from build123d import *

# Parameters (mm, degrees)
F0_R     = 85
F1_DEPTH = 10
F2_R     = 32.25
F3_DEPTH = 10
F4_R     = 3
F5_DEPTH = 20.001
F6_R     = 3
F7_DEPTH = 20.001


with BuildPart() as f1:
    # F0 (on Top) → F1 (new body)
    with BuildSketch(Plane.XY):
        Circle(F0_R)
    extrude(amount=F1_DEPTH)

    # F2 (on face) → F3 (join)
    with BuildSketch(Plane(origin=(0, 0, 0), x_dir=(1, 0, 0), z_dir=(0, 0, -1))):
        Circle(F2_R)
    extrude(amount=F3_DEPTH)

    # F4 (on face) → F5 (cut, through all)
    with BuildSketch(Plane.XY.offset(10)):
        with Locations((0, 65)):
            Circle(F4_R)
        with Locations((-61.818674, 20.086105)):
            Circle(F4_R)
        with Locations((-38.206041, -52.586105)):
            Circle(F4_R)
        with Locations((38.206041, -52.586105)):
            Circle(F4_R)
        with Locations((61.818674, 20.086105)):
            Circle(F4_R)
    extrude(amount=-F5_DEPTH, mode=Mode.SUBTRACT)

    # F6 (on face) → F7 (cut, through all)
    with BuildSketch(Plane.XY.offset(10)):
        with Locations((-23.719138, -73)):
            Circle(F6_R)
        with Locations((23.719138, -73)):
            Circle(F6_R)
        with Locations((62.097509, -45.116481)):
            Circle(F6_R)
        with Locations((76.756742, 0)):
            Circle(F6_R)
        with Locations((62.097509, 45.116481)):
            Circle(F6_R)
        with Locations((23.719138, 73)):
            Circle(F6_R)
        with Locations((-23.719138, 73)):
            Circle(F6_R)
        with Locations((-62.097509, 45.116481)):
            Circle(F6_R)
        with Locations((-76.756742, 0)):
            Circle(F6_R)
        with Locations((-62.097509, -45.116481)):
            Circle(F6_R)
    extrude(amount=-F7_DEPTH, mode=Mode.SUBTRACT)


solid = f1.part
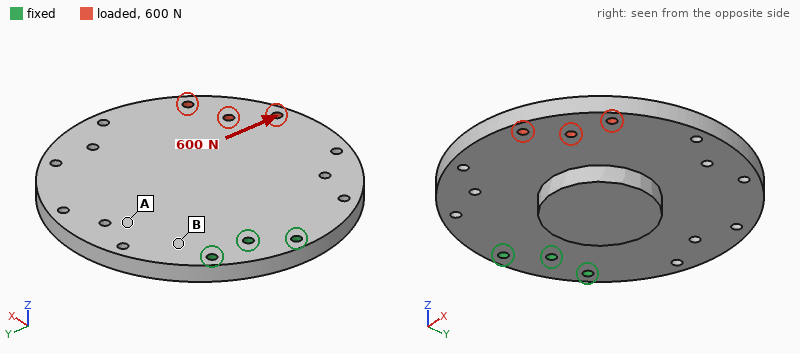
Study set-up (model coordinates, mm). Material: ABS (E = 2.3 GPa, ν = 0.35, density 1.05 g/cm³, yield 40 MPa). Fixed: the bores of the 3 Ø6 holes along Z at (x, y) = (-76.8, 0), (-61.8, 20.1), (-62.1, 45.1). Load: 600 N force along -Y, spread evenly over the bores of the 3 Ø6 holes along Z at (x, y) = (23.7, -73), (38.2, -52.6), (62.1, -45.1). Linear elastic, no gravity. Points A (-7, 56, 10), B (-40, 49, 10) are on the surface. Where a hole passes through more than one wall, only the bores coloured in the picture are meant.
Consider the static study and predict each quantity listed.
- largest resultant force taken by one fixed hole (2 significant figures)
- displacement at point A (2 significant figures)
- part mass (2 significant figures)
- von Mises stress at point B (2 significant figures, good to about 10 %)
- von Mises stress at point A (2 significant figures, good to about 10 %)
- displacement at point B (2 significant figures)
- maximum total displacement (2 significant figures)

1.2 kN
0.23 mm
270 g
2.8 MPa
0.87 MPa
0.10 mm
0.55 mm
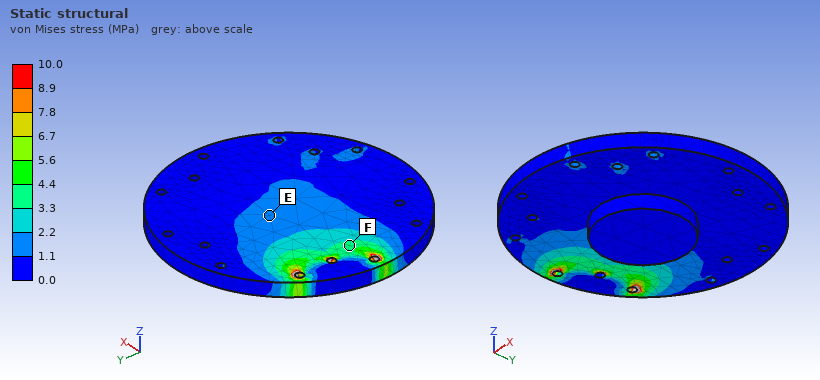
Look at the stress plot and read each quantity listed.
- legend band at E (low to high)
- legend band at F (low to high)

1.1 to 2.2 MPa
3.3 to 4.4 MPa
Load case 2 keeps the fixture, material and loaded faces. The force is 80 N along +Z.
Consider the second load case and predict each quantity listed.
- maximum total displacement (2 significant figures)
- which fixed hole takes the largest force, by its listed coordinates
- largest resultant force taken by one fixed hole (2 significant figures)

2.8 mm
(-61.8, 20.1)
200 N
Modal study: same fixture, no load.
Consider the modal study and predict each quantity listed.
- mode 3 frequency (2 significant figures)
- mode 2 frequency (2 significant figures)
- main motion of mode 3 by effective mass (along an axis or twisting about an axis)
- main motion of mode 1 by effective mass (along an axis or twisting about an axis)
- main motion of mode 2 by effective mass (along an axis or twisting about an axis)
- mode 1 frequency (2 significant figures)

480 Hz
250 Hz
along Y
along Z
twisting about X
100 Hz
